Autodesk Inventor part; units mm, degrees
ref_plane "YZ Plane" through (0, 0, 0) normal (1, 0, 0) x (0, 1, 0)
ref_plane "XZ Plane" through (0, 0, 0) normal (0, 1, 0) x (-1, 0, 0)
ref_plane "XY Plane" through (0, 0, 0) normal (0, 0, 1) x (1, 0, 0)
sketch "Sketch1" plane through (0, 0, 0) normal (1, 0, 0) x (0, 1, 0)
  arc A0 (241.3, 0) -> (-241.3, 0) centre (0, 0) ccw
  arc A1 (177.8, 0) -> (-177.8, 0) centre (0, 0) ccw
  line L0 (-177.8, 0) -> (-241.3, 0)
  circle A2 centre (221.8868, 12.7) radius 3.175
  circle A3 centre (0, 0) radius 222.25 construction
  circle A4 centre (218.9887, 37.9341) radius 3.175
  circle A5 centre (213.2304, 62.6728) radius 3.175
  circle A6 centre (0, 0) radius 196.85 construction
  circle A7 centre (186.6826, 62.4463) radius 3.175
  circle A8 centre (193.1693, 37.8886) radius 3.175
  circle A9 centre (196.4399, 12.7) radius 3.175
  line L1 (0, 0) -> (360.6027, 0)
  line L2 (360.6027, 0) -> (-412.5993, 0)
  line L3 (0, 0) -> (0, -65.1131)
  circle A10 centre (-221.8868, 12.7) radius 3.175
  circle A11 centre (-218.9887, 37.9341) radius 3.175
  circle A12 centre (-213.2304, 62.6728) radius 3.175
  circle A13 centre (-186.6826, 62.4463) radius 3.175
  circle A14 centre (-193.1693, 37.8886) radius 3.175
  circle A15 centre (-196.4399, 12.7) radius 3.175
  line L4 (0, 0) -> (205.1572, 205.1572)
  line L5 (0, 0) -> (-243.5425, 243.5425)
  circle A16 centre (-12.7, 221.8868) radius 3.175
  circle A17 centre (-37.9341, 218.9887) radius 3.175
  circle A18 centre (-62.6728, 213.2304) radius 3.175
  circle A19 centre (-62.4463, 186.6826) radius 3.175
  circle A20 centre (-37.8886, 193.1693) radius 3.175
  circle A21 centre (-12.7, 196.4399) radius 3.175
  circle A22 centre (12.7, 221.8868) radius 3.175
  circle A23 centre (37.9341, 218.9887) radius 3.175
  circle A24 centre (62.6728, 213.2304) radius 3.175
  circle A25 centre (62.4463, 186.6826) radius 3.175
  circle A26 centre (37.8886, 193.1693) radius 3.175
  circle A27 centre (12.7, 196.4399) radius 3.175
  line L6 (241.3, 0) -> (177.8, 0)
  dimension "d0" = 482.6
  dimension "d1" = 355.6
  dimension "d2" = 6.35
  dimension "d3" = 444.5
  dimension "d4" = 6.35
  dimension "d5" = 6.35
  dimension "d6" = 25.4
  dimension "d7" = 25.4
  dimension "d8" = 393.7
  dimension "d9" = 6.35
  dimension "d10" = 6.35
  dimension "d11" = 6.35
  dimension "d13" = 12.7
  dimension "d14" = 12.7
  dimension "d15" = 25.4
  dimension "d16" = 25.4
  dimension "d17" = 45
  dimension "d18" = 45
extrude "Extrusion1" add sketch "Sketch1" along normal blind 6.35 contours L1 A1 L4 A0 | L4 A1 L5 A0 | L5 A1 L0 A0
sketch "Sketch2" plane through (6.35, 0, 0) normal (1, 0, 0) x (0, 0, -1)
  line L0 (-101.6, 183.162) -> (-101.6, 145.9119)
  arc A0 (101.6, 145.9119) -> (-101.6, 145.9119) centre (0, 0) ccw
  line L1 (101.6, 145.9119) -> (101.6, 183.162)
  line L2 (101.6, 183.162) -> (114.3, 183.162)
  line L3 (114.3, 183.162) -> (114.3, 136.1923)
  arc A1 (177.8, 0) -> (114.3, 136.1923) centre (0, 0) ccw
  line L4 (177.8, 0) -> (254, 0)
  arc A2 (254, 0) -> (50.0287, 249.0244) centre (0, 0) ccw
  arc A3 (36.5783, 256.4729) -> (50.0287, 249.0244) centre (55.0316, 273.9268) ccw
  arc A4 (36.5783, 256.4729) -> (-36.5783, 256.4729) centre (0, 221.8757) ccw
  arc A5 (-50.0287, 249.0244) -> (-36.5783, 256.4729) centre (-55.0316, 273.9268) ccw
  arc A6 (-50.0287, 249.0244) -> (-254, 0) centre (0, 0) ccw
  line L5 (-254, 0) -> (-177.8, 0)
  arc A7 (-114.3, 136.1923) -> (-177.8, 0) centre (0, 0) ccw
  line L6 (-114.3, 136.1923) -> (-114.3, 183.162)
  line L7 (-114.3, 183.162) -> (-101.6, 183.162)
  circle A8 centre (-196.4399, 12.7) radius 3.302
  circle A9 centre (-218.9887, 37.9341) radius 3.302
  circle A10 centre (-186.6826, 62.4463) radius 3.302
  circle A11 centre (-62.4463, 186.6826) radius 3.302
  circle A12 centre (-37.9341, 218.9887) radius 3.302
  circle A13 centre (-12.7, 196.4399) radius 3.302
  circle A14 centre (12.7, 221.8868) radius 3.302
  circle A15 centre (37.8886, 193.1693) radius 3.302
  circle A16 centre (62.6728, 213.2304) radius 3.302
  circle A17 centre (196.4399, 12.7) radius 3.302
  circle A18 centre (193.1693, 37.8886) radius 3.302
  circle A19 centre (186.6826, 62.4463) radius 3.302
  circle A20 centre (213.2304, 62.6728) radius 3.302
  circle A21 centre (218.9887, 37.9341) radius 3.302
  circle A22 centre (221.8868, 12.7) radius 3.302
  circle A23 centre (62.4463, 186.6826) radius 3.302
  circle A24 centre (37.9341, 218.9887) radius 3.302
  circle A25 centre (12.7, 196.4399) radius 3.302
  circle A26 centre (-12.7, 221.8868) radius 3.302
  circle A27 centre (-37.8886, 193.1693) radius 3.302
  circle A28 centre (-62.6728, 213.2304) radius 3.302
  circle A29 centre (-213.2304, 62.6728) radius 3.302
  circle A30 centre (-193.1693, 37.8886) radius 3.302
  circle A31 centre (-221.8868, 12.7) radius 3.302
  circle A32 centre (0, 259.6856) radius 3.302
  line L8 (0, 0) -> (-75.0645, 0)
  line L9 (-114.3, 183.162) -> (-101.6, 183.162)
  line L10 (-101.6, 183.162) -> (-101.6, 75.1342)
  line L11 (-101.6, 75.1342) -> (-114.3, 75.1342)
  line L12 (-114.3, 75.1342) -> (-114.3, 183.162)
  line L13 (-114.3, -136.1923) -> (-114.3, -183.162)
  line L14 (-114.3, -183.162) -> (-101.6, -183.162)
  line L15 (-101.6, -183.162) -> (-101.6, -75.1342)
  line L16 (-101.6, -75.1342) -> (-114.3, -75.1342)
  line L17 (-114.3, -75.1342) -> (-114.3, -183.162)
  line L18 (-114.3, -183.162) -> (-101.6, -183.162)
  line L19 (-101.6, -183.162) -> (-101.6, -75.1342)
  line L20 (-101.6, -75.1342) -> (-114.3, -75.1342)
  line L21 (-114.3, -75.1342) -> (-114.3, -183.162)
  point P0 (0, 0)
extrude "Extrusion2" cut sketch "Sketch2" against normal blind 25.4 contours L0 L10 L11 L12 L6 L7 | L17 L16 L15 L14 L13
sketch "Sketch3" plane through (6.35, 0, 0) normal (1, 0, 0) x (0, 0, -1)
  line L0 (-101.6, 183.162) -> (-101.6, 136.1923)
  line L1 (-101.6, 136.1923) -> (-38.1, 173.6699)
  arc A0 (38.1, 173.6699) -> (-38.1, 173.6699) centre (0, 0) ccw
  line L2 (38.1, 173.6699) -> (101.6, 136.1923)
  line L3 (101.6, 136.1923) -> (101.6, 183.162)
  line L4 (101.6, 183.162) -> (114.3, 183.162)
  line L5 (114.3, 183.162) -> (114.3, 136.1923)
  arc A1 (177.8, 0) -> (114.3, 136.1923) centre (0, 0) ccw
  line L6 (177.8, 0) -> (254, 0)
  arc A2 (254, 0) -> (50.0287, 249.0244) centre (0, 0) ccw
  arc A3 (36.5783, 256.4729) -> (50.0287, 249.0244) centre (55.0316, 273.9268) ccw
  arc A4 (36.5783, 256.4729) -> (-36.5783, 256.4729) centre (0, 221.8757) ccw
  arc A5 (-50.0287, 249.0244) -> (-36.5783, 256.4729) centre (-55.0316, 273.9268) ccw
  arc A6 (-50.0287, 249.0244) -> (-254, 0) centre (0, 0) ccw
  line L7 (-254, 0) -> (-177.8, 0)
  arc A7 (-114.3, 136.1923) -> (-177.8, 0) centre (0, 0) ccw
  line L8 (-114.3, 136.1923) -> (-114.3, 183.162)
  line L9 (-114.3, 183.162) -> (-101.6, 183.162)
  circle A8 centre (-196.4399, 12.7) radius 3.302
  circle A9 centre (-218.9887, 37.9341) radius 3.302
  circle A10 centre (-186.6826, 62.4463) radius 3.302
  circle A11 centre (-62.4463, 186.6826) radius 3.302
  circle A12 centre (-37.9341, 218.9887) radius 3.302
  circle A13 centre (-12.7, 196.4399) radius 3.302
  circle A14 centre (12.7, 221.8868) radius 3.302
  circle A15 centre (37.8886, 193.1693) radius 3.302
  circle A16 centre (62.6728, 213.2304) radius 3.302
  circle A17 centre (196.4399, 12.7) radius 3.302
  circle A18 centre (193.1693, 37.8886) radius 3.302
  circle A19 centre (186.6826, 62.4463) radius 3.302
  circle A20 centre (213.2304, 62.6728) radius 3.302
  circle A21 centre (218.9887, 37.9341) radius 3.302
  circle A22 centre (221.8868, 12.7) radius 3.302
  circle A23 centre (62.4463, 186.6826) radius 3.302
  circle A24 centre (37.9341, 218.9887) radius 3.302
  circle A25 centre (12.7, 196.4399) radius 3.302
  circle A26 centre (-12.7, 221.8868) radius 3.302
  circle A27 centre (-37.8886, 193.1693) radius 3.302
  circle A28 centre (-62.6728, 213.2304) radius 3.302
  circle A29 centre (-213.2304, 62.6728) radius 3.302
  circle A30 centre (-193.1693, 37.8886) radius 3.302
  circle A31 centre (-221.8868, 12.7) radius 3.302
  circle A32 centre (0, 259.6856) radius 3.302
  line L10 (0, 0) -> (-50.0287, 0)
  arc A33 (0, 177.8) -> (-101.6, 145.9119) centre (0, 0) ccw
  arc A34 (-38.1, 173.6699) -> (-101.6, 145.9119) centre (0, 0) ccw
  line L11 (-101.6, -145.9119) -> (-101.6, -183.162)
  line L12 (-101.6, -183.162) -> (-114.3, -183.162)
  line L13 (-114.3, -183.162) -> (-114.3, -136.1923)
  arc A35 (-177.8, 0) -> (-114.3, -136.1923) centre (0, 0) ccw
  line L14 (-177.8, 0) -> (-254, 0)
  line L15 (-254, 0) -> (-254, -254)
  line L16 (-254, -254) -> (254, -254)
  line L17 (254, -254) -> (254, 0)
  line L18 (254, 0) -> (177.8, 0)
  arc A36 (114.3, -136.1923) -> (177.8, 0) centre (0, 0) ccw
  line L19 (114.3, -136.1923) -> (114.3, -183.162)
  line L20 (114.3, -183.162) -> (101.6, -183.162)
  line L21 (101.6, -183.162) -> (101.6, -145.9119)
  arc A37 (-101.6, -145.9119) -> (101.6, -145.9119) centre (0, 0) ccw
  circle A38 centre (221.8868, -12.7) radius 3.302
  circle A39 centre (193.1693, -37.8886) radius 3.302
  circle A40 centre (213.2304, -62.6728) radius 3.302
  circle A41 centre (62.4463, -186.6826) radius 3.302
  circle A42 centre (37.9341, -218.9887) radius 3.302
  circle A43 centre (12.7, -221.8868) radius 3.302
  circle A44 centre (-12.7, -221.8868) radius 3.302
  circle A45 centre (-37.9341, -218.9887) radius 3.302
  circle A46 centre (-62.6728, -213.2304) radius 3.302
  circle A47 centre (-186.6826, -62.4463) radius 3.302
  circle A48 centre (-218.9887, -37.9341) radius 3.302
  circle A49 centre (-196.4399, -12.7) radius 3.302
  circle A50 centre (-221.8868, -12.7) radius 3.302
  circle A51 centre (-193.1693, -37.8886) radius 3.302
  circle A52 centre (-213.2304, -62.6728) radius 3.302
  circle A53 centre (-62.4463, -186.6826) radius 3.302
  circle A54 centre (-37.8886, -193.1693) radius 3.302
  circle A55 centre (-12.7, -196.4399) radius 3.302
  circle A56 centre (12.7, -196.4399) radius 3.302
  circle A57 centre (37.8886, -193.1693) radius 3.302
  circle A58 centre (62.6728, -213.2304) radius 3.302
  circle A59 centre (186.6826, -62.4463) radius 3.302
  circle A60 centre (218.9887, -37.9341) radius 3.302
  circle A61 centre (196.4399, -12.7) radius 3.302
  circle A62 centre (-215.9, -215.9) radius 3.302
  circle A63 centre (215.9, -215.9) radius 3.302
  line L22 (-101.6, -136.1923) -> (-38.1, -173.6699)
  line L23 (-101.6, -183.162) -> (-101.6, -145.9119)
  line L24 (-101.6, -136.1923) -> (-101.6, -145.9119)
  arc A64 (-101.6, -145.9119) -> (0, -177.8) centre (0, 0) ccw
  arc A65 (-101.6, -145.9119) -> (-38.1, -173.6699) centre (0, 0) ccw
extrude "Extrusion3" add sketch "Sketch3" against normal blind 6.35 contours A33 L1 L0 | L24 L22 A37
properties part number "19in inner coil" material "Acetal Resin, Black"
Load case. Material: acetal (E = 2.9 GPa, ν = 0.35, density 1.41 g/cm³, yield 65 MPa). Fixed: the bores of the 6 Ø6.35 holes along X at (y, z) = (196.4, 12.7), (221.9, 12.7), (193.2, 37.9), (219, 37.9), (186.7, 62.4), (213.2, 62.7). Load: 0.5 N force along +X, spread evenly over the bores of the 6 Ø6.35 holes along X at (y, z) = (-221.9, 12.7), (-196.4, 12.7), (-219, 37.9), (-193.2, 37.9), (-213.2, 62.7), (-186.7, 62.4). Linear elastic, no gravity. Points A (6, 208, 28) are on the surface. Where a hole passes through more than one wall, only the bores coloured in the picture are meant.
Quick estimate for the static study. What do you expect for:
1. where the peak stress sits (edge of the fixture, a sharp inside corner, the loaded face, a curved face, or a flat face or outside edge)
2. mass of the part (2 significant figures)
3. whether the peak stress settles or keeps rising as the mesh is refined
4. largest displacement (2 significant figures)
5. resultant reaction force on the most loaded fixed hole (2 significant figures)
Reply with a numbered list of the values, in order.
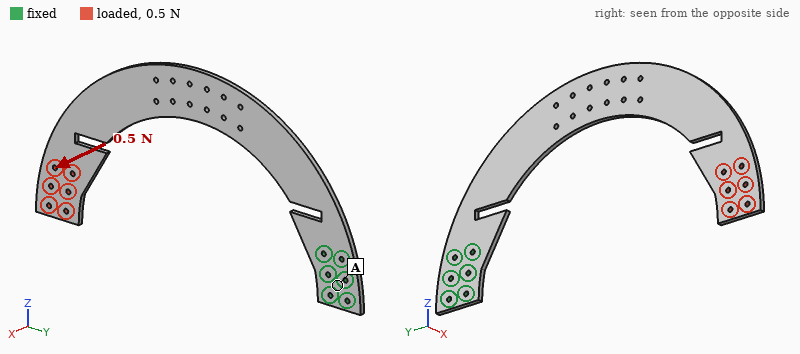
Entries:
1. a sharp inside corner
2. 370 g
3. keeps rising
4. 6.0 mm
5. 6.8 N
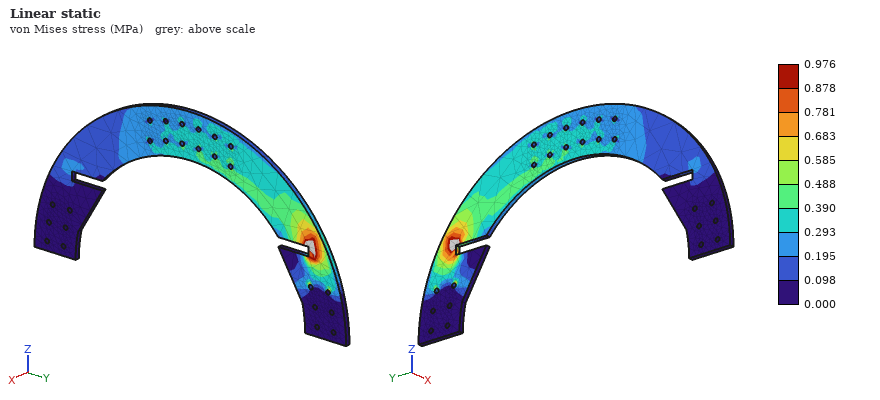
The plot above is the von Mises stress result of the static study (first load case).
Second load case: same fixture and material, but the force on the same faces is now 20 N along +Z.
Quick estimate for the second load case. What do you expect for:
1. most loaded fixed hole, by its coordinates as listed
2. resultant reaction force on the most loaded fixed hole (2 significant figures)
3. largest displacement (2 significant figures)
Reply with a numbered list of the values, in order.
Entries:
1. (186.7, 62.4)
2. 180 N
3. 6.4 mm
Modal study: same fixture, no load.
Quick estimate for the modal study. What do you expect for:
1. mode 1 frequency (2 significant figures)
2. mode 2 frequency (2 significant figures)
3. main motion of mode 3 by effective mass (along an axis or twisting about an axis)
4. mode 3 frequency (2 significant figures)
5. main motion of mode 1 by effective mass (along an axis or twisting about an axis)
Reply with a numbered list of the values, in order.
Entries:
1. 4.7 Hz
2. 15 Hz
3. along Z
4. 26 Hz
5. along X
